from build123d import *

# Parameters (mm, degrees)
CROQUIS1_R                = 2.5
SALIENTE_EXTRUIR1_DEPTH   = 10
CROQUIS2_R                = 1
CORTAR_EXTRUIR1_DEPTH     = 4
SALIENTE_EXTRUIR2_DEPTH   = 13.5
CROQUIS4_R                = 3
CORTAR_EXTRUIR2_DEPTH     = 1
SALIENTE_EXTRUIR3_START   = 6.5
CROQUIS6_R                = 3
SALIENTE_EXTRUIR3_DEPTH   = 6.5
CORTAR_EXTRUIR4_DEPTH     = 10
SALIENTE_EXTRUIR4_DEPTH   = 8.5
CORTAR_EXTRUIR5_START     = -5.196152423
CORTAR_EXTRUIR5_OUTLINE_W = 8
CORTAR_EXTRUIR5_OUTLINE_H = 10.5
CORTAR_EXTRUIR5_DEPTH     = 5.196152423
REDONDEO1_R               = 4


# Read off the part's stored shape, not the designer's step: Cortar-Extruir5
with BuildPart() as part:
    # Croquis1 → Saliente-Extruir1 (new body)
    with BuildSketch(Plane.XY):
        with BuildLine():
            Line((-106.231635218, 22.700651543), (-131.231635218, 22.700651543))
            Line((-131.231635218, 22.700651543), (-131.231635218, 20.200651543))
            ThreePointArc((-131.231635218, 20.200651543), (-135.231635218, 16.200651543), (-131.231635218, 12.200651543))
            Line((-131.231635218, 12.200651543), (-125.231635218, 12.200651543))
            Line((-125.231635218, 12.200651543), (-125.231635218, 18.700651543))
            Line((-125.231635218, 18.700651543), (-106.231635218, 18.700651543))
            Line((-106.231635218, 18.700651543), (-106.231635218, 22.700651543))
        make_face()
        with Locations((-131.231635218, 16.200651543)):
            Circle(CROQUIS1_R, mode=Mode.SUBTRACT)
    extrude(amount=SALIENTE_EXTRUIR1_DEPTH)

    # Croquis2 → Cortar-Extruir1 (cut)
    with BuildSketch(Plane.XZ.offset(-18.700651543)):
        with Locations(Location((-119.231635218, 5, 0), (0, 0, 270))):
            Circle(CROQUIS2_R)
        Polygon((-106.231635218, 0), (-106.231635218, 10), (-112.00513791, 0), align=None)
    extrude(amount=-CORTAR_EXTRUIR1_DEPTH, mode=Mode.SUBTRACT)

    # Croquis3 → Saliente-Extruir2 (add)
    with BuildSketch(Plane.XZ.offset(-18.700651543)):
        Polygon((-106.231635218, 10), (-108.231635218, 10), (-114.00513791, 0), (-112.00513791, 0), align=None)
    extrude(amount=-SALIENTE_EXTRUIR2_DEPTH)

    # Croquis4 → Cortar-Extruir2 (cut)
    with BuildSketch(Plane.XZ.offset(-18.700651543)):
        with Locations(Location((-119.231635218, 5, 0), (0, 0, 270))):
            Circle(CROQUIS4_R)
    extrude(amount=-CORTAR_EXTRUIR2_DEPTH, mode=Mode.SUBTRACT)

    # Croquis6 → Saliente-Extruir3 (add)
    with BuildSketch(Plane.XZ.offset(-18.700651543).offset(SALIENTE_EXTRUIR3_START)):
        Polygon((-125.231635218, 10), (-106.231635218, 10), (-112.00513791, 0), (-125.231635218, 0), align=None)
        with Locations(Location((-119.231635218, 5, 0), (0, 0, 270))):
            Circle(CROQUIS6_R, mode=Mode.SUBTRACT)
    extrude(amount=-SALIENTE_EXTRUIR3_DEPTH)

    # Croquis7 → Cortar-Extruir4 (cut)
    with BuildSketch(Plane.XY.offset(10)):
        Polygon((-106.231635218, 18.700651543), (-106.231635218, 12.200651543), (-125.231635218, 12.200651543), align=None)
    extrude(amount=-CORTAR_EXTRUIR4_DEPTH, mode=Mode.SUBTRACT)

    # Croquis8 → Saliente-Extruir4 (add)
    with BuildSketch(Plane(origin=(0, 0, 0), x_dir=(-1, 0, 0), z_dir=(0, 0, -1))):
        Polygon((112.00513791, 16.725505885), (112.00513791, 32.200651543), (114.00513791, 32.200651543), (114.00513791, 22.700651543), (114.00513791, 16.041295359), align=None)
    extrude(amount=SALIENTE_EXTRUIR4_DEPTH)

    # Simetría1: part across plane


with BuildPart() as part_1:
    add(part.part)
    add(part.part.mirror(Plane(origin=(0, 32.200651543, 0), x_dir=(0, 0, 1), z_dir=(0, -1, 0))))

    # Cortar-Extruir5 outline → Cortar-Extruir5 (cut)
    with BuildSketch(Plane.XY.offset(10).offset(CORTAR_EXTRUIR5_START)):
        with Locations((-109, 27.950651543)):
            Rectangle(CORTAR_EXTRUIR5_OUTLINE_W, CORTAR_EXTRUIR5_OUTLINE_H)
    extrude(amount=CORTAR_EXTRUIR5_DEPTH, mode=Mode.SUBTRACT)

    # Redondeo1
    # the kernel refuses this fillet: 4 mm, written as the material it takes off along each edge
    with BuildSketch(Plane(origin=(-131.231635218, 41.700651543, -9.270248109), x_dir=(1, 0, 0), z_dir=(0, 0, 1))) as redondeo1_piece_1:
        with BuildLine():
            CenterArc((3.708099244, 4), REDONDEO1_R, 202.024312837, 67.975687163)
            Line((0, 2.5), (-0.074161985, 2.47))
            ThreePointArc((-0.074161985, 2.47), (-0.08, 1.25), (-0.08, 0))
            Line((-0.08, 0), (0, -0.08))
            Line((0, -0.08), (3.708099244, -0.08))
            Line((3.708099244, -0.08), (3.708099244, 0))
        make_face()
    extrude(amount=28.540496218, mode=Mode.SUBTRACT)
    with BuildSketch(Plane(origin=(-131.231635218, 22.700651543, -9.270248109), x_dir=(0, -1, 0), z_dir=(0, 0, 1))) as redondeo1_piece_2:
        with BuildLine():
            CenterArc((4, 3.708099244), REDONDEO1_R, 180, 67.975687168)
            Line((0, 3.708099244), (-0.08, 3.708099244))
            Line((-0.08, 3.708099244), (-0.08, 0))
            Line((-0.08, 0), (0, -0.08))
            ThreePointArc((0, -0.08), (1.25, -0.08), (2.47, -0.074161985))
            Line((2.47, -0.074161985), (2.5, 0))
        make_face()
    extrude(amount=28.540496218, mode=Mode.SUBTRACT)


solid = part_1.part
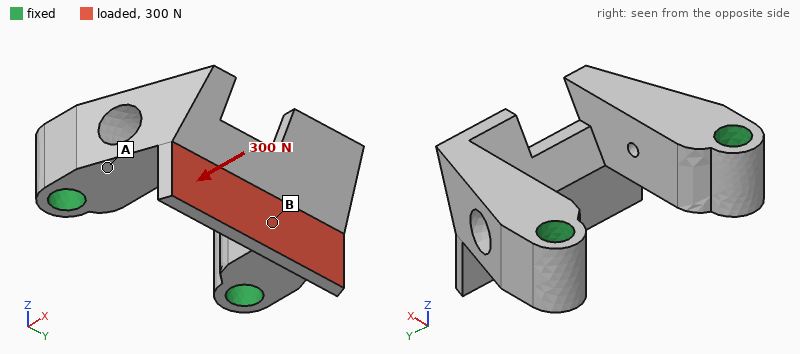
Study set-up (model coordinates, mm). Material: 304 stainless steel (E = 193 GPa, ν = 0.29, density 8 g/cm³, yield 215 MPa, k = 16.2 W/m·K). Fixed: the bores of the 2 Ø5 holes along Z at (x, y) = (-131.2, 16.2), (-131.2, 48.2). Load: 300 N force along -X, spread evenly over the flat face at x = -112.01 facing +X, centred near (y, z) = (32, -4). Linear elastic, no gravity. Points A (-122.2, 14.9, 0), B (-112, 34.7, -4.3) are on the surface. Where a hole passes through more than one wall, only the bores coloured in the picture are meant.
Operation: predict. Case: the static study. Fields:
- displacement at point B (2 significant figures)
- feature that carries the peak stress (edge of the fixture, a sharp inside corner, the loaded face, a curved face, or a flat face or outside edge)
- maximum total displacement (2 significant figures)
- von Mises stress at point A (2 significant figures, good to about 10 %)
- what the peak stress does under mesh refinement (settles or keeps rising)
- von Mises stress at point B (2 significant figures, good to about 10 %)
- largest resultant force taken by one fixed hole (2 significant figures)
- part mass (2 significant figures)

13 µm
a sharp inside corner
22 µm
11 MPa
keeps rising
25 MPa
160 N
34 g
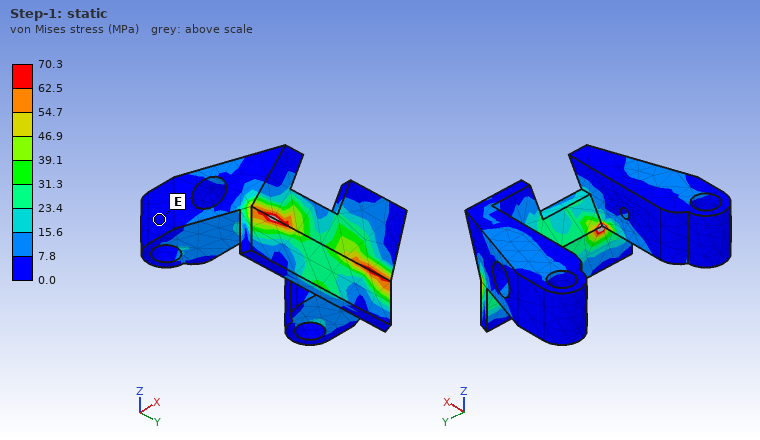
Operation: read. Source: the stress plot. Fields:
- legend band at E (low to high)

0.0 to 7.8 MPa
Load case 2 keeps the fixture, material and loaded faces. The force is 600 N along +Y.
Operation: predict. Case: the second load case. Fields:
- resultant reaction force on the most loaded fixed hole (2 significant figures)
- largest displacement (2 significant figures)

330 N
12 µm
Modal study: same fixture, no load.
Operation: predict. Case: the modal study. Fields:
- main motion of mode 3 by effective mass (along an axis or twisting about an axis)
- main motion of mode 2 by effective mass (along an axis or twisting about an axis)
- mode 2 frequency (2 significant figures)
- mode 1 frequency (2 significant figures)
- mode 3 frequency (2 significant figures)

along Z
along Y
12 kHz
11 kHz
14 kHz
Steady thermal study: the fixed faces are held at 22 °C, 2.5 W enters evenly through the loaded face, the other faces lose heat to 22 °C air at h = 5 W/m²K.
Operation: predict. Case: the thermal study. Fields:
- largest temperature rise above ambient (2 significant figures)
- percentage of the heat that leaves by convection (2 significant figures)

42 K
8.1 %
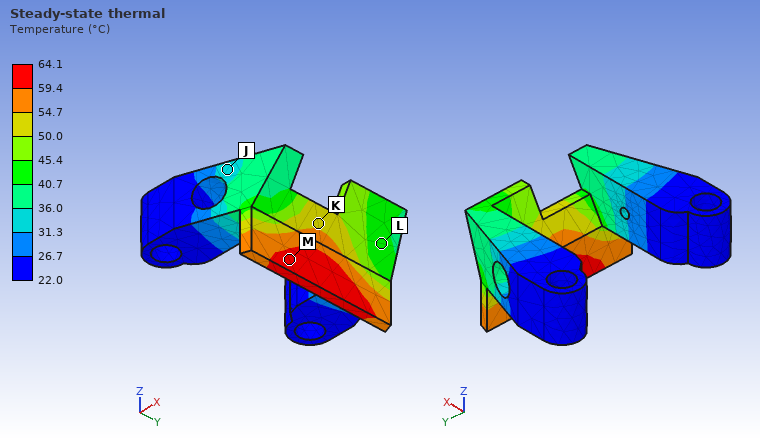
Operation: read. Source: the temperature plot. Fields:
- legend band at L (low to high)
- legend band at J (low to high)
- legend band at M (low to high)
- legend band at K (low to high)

40.7 to 45.4 °C
31.3 to 36.0 °C
59.4 to 64.1 °C
50.0 to 54.7 °C
